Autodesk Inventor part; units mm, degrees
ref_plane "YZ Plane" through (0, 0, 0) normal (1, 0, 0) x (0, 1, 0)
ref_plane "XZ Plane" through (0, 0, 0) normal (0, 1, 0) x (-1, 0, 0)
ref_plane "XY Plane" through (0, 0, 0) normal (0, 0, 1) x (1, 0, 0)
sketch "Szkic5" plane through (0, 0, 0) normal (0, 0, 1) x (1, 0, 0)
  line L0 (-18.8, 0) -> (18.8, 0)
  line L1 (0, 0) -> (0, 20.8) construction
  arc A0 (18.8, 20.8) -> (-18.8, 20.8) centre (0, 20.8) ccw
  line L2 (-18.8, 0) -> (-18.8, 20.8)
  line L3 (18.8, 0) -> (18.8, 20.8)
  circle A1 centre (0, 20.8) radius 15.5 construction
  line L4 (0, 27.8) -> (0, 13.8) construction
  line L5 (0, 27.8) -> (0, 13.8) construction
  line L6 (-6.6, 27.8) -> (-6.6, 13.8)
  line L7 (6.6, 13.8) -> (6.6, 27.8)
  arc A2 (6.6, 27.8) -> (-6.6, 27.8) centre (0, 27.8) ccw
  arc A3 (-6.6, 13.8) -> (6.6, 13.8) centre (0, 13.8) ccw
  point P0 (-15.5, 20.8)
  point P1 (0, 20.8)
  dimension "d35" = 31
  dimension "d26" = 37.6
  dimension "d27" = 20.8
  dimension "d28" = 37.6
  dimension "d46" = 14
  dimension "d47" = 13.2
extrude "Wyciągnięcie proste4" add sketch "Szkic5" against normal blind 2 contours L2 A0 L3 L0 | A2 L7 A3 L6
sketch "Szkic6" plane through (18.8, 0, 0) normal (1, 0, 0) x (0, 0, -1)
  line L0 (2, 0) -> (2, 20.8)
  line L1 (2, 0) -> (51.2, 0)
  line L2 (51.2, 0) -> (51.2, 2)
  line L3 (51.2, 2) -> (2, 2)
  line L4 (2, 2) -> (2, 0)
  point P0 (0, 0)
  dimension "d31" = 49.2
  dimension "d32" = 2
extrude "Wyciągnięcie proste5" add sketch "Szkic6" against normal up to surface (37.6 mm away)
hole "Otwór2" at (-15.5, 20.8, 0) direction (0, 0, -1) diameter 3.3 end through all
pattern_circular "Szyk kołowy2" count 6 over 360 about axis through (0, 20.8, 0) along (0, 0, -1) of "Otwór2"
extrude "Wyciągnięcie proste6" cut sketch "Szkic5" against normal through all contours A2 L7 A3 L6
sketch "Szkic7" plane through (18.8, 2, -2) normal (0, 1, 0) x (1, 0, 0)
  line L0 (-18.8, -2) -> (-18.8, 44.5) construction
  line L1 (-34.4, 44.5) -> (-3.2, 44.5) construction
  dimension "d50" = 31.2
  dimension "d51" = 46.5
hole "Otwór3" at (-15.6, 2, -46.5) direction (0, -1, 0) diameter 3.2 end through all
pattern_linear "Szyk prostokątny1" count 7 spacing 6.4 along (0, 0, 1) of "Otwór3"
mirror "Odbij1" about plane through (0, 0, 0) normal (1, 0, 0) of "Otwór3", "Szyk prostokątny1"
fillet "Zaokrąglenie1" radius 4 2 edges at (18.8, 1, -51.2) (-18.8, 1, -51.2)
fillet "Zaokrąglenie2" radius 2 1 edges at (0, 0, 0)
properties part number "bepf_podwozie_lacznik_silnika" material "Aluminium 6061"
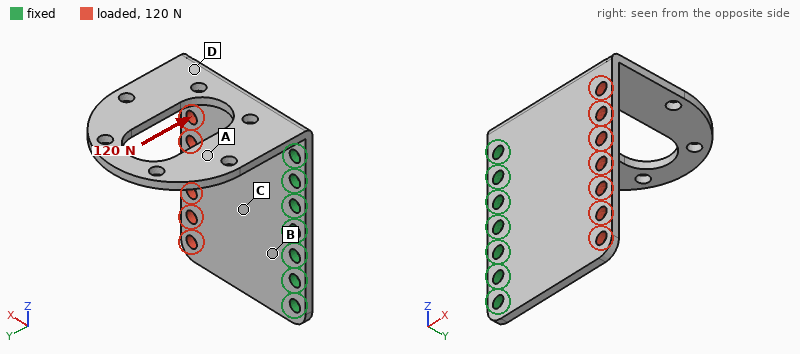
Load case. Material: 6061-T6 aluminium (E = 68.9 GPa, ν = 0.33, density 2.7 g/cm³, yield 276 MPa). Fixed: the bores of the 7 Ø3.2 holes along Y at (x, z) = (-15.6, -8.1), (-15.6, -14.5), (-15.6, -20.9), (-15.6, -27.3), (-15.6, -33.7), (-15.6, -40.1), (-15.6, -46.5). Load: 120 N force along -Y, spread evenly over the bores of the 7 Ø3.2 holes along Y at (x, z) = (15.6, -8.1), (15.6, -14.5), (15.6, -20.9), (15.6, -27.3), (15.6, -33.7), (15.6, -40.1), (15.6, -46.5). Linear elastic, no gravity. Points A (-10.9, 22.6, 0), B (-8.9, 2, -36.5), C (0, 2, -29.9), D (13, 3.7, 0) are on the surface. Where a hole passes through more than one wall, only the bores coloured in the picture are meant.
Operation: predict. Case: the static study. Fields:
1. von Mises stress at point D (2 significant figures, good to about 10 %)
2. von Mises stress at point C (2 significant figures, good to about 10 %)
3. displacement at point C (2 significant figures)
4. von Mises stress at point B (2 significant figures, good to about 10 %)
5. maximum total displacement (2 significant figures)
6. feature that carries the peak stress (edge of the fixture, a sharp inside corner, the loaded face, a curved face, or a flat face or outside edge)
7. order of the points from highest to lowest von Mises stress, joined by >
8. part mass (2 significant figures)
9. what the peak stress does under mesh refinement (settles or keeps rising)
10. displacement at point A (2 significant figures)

21 MPa
39 MPa
0.11 mm
68 MPa
0.44 mm
edge of the fixture
B > C > D > A
14 g
keeps rising
0.15 mm
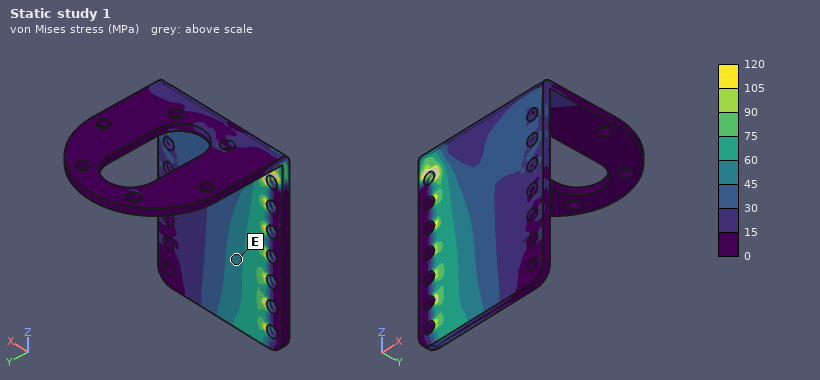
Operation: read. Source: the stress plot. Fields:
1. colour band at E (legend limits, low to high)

45 to 60 MPa
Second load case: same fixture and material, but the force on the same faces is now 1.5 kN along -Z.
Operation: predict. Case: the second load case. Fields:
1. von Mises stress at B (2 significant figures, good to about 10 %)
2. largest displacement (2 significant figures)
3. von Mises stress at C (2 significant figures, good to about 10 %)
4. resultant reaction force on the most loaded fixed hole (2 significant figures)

37 MPa
42 µm
40 MPa
960 N
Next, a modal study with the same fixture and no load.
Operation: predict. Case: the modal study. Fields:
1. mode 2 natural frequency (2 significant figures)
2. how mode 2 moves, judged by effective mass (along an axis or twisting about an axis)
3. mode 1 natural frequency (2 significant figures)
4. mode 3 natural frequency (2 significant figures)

1200 Hz
along Y
910 Hz
2200 Hz
